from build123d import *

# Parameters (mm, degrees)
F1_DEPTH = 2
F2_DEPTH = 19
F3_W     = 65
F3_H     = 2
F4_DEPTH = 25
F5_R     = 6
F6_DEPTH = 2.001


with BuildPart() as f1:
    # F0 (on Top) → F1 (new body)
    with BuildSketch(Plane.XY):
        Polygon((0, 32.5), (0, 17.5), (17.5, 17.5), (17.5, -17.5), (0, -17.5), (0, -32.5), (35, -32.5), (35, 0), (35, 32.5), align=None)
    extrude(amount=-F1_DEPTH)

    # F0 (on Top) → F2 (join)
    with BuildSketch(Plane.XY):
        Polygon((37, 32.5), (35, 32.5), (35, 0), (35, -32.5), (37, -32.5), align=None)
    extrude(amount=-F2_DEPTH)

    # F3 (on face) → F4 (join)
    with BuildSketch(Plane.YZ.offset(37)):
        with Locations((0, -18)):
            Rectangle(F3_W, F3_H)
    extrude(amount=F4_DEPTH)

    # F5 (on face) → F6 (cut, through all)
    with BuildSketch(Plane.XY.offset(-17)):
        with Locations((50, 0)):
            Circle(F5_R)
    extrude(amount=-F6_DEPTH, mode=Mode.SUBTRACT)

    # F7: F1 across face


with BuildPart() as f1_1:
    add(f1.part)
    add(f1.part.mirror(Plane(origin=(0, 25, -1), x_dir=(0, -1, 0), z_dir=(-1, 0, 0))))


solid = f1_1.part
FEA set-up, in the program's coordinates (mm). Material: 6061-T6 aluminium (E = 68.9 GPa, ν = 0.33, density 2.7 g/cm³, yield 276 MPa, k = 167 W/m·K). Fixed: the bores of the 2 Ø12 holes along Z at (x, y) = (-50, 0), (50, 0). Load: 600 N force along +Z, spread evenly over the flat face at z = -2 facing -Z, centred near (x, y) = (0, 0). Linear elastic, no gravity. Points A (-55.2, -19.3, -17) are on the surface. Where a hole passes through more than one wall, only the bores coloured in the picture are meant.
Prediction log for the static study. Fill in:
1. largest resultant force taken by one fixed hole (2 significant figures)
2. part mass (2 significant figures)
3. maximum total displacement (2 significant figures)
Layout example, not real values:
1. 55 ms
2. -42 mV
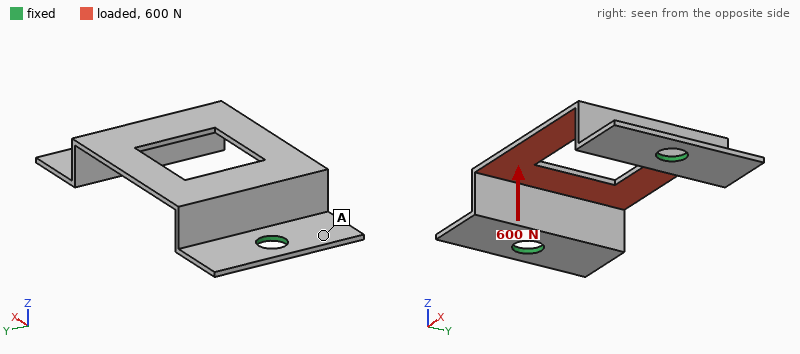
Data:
1. 430 N
2. 48 g
3. 0.32 mm
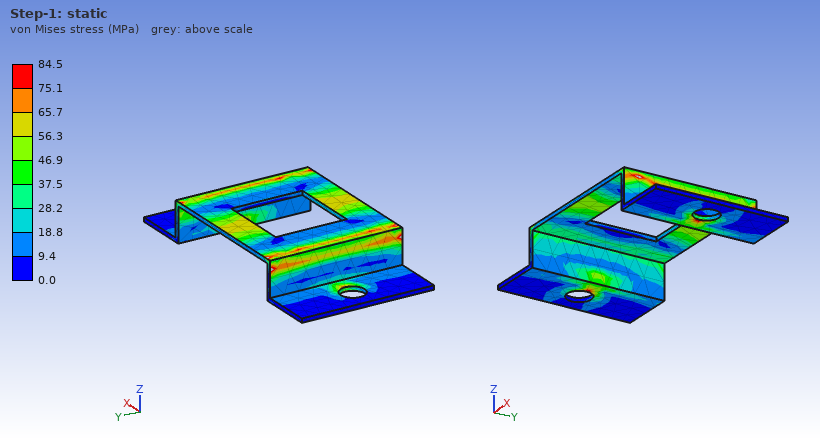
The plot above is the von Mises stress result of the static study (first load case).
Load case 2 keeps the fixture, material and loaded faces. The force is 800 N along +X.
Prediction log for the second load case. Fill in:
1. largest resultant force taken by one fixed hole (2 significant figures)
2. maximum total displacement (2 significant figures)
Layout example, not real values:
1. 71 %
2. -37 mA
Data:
1. 410 N
2. 0.36 mm
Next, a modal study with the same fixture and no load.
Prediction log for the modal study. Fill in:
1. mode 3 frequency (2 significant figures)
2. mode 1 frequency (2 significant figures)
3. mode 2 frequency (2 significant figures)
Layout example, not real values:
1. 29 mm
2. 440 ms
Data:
1. 1600 Hz
2. 1200 Hz
3. 1600 Hz
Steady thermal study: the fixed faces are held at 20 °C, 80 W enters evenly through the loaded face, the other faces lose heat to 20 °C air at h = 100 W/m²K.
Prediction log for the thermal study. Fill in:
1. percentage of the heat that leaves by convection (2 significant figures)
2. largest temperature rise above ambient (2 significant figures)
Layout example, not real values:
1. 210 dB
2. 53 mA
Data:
1. 50 %
2. 64 K
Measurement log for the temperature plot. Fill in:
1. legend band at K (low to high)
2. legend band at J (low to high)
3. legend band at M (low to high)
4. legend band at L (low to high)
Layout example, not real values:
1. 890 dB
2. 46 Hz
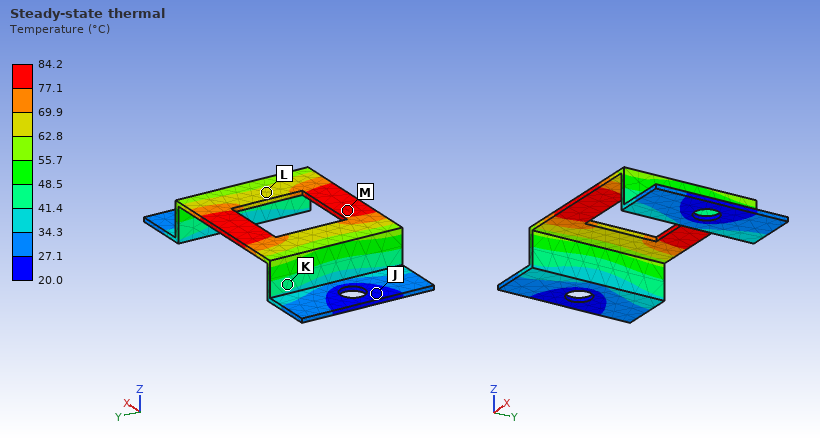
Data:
1. 41.4 to 48.5 °C
2. 20.0 to 27.1 °C
3. 77.1 to 84.2 °C
4. 62.8 to 69.9 °C
